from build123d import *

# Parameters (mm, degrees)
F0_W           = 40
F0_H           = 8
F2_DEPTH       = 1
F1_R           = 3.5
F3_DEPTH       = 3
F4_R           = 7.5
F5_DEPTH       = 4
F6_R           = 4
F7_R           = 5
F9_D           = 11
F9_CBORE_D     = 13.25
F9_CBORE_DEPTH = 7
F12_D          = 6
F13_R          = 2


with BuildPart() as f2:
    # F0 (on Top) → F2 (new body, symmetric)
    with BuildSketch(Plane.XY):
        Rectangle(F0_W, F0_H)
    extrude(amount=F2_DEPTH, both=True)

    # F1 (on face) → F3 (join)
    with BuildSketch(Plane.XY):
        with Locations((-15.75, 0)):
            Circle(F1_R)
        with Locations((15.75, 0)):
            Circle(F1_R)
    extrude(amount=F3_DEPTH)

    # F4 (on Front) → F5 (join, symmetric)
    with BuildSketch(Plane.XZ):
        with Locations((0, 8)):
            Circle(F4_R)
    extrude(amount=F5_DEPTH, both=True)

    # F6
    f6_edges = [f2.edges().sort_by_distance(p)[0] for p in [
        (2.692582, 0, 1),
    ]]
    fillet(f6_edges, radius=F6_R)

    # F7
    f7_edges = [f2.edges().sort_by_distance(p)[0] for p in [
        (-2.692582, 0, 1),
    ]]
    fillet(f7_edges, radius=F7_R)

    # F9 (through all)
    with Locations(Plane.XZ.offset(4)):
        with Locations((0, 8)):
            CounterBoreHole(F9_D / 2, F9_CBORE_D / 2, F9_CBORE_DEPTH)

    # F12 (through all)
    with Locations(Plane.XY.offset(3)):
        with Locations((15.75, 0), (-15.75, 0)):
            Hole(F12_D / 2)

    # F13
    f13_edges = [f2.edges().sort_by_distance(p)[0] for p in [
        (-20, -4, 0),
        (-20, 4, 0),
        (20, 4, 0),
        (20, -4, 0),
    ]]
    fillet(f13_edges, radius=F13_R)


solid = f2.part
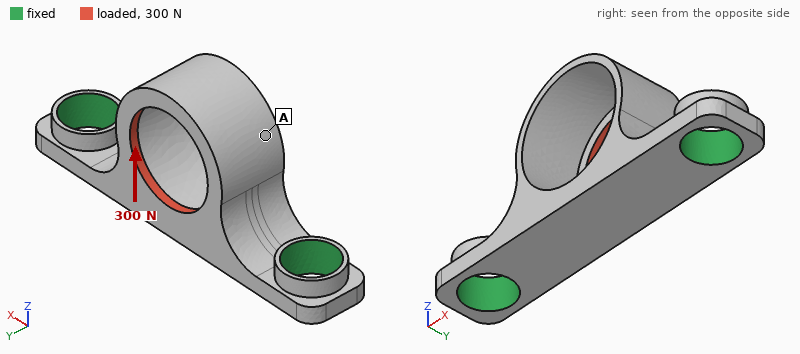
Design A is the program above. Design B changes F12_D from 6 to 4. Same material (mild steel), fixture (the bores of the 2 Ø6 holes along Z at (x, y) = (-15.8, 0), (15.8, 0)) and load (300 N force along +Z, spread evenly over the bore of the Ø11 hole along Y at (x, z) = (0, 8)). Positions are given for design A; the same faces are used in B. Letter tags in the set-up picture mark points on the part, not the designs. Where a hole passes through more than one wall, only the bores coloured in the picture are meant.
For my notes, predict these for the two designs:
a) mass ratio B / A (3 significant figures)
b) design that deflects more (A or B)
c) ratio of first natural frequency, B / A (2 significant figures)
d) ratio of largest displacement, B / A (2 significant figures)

1.11
B
0.92
1.2
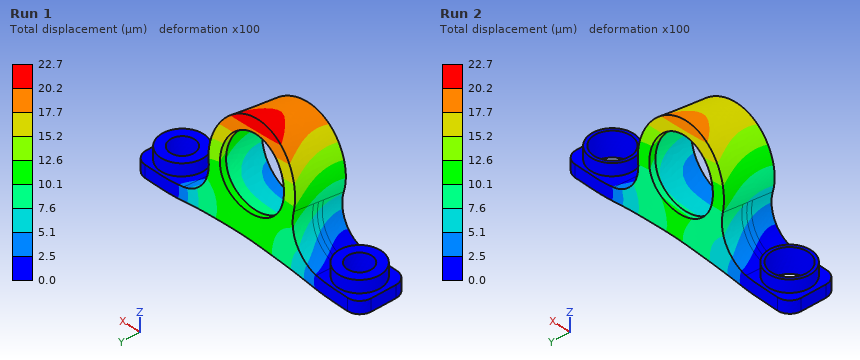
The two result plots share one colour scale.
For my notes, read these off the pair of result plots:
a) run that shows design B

Run 1
